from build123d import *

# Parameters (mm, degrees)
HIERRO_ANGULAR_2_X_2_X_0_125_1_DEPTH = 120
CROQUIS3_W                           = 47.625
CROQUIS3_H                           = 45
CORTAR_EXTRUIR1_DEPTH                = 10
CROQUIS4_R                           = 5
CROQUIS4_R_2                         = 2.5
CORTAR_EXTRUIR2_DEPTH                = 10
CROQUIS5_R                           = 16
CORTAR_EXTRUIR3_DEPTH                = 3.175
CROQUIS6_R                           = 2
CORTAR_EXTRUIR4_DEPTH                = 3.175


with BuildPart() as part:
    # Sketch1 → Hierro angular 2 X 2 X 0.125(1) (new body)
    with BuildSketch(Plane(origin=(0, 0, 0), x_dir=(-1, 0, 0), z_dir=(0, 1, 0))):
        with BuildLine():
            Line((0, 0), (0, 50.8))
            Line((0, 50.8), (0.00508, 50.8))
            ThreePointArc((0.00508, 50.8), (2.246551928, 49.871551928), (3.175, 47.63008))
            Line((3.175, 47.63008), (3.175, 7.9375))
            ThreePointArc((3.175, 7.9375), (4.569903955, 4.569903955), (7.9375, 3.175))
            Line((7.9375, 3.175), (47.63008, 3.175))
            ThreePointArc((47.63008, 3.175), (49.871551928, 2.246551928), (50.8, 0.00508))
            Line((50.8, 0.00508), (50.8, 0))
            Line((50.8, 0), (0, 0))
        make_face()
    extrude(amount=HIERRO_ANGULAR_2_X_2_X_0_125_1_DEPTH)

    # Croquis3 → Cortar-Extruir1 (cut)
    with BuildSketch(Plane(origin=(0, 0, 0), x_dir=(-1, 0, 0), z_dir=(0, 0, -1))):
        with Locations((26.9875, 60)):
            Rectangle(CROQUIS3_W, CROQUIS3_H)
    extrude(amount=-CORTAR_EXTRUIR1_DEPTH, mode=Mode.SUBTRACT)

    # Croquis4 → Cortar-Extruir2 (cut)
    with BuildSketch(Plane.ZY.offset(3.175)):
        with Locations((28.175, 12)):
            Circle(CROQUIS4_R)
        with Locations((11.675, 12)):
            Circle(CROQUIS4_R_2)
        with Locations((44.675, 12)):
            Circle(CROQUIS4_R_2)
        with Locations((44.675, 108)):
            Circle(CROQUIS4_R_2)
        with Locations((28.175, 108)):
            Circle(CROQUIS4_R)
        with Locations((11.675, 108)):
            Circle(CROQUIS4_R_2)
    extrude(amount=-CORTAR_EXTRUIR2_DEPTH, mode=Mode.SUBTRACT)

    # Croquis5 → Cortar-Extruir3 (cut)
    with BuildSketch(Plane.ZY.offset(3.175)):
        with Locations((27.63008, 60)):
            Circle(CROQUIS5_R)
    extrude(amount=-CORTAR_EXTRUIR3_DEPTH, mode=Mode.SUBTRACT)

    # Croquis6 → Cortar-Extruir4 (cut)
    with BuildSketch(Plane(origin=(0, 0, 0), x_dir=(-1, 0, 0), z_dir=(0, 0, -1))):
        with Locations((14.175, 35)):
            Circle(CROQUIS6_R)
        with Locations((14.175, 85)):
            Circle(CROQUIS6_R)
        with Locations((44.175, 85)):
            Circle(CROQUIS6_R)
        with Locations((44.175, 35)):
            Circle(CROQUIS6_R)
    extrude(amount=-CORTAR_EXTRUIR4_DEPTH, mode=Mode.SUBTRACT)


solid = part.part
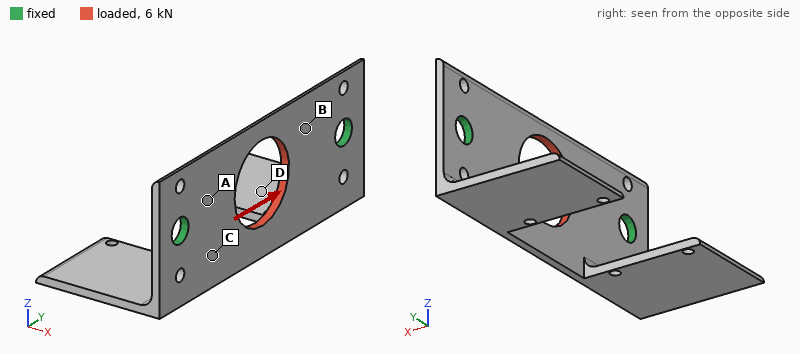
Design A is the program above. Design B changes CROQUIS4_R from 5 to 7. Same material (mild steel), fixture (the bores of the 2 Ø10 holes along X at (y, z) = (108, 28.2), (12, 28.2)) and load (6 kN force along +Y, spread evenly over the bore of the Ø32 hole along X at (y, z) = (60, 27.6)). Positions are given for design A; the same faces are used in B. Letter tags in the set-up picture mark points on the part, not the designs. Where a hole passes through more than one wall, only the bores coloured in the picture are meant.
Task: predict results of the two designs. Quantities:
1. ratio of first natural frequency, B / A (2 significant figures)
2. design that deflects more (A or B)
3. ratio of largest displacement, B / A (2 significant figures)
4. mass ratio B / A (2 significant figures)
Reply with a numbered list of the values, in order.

1. 1.1
2. A
3. 0.91
4. 0.98
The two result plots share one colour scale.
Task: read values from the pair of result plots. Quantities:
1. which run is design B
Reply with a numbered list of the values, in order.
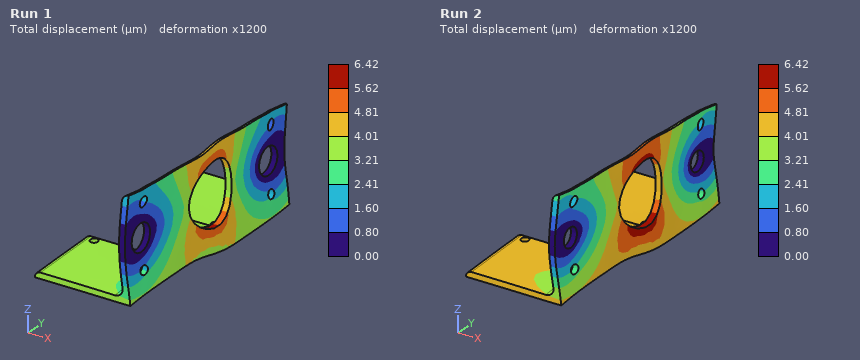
1. Run 1
